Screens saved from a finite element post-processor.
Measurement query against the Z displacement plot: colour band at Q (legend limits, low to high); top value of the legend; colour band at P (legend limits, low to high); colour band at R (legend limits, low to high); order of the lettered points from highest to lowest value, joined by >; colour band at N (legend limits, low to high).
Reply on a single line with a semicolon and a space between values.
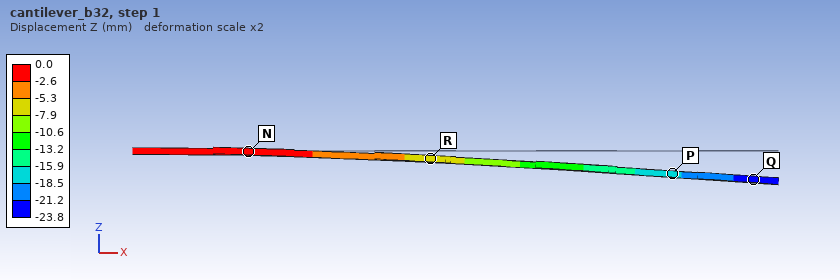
-23.8 to -21.2 mm; 0.0 mm; -18.5 to -15.9 mm; -7.9 to -5.3 mm; N > R > P > Q; -2.6 to 0.0 mm
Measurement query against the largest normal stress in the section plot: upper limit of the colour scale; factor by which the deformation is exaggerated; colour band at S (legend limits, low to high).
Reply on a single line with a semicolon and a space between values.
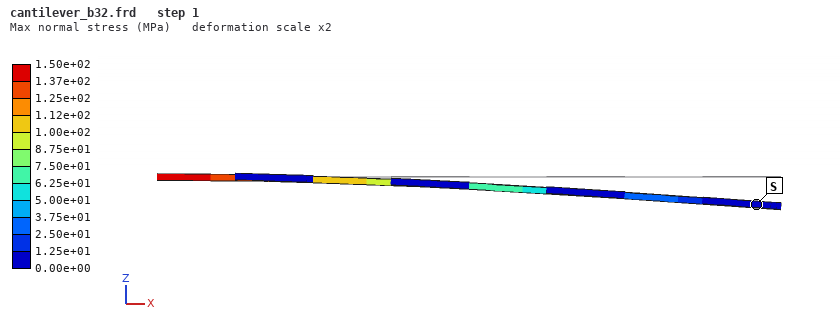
1.50e+02 MPa; 2; 0.00e+00 to 1.25e+01 MPa
